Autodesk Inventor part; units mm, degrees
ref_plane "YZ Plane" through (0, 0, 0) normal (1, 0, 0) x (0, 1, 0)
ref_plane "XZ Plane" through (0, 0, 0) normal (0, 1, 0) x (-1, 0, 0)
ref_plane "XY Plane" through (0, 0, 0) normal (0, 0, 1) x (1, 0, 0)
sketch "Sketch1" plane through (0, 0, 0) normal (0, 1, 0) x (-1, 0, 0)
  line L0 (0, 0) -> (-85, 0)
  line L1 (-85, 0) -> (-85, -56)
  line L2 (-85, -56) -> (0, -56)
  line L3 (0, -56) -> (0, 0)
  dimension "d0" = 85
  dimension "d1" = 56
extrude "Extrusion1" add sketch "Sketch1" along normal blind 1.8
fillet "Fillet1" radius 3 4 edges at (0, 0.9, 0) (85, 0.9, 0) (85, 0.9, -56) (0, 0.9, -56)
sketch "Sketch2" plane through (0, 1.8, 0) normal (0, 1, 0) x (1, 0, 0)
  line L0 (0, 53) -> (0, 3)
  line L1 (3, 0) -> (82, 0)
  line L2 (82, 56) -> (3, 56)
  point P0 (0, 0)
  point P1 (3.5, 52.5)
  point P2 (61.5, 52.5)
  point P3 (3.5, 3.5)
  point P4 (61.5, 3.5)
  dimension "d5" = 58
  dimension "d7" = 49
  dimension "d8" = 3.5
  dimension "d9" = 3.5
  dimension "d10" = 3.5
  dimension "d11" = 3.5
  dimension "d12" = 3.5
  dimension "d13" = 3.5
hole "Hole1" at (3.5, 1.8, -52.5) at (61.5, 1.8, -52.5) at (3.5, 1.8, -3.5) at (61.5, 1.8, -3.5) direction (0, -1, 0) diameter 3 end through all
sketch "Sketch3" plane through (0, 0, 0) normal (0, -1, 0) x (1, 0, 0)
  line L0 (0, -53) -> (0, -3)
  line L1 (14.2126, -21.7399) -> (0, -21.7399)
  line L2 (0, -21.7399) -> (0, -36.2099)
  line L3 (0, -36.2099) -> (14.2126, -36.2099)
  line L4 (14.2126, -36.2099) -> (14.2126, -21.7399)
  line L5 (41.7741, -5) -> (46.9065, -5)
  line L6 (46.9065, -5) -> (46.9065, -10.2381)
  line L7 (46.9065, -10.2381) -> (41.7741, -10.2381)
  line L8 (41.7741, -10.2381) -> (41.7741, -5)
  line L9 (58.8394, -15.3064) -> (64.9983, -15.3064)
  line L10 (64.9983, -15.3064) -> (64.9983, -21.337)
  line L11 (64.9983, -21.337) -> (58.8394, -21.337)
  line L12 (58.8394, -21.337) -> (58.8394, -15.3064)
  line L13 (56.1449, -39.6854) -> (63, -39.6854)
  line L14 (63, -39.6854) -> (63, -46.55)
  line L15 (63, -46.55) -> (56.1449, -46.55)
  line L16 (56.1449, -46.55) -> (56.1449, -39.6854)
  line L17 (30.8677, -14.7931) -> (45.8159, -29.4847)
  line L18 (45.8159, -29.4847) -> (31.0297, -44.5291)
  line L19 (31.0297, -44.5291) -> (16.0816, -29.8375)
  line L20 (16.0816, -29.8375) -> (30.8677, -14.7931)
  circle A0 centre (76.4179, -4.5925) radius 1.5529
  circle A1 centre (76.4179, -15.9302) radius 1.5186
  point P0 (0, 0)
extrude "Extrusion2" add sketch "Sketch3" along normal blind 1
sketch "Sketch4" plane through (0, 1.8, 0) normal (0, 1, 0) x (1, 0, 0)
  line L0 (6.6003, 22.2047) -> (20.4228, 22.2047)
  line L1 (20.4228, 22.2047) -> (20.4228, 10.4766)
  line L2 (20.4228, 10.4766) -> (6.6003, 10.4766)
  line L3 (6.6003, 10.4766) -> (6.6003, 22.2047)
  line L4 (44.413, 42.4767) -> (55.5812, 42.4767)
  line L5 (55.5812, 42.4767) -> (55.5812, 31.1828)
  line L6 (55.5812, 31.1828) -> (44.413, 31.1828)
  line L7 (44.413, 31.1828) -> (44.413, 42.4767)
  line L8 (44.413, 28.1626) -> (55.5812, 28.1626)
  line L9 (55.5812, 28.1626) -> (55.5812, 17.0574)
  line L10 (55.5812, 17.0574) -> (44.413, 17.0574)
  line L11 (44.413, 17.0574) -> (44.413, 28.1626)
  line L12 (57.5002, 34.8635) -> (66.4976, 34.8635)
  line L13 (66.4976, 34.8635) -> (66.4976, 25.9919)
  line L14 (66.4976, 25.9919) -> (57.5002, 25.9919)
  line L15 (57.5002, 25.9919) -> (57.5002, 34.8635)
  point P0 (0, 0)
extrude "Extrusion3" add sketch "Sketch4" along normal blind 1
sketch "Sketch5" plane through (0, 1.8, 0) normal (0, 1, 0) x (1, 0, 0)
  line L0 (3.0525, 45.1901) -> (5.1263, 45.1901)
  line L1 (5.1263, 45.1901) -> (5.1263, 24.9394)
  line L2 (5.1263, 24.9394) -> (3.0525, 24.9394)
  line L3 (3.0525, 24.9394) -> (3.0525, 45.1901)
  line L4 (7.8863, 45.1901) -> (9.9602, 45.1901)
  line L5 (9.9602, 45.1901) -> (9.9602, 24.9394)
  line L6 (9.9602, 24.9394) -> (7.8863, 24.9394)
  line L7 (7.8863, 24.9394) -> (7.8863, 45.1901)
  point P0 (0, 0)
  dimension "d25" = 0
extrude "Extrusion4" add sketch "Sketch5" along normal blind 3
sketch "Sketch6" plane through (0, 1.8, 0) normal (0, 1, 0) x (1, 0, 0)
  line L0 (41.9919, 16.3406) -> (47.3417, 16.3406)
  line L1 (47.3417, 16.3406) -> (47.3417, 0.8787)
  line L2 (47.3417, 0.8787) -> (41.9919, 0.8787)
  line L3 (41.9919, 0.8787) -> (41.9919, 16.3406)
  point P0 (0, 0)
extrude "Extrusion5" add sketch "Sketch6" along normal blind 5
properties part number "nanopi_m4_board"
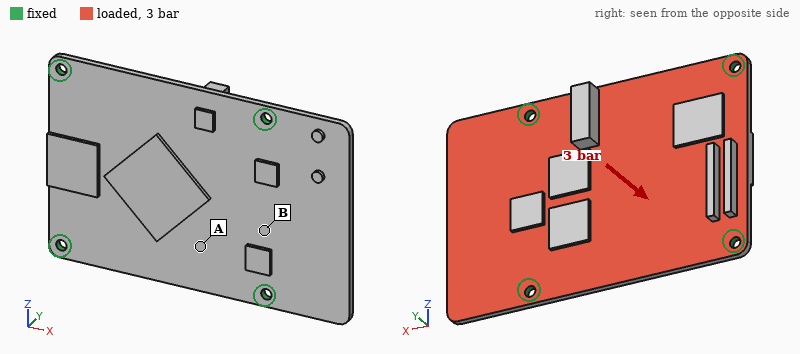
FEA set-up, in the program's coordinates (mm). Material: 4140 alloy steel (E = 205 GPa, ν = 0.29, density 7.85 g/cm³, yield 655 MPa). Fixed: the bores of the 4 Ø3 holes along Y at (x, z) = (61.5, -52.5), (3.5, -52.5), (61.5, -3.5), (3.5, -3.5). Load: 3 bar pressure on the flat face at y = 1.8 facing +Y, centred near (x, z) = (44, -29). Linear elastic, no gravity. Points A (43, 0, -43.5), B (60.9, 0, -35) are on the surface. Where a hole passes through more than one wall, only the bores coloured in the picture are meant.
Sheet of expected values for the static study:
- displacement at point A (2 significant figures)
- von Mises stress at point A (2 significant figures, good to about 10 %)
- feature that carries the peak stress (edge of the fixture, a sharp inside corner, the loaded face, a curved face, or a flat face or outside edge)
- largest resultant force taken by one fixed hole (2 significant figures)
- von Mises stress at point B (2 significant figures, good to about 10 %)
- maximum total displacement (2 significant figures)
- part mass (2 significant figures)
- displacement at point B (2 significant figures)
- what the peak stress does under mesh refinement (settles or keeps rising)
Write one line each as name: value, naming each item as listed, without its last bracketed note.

displacement at point A: 0.067 mm
von Mises stress at point A: 35 MPa
feature that carries the peak stress: edge of the fixture
largest resultant force taken by one fixed hole: 410 N
von Mises stress at point B: 82 MPa
maximum total displacement: 0.16 mm
part mass: 82 g
displacement at point B: 0.054 mm
what the peak stress does under mesh refinement: keeps rising
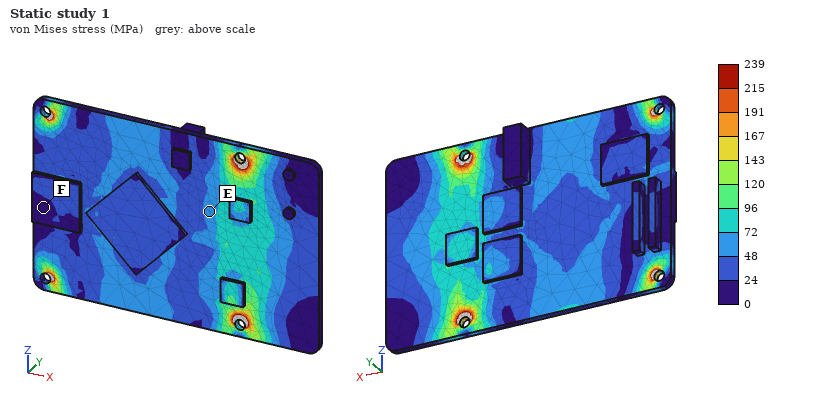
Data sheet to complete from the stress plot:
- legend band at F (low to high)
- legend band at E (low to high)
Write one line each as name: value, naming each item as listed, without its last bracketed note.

legend band at F: 0 to 24 MPa
legend band at E: 48 to 72 MPa
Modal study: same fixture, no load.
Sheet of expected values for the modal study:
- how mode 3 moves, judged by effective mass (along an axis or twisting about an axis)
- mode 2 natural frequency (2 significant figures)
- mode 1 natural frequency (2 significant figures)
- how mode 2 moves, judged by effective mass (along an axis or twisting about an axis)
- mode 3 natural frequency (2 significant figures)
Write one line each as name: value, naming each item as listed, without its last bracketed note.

how mode 3 moves, judged by effective mass: twisting about X
mode 2 natural frequency: 2300 Hz
mode 1 natural frequency: 2000 Hz
how mode 2 moves, judged by effective mass: along Y
mode 3 natural frequency: 3600 Hz
